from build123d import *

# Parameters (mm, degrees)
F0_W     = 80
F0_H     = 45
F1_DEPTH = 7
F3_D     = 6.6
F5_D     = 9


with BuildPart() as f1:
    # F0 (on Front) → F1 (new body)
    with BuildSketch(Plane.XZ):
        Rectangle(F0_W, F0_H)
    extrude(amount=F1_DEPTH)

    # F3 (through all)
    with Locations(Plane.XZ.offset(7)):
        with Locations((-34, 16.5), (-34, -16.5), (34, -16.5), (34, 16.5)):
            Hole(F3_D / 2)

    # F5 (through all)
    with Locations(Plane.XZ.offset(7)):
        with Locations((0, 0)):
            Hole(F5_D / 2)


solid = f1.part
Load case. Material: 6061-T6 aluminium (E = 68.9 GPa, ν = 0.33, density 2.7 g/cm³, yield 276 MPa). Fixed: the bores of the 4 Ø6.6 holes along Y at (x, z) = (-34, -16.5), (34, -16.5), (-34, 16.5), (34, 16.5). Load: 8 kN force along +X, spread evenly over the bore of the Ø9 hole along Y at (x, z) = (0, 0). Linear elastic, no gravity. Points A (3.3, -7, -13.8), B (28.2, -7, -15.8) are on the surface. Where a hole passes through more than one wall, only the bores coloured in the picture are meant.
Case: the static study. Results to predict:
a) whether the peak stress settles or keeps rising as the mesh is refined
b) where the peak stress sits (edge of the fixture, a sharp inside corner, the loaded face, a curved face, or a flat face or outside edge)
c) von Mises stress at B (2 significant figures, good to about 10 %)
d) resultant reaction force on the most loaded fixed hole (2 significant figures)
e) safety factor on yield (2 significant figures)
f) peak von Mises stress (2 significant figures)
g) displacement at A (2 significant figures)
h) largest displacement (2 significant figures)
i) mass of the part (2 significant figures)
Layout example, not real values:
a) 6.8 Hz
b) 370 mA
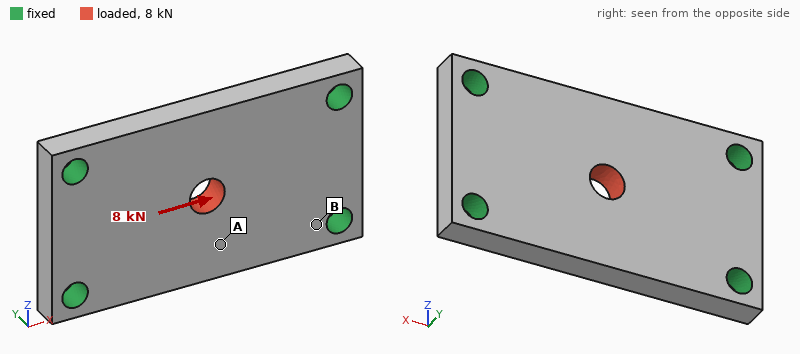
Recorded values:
a) settles
b) the loaded face
c) 23 MPa
d) 2.1 kN
e) 4.0
f) 69 MPa
g) 5.0 µm
h) 11 µm
i) 64 g
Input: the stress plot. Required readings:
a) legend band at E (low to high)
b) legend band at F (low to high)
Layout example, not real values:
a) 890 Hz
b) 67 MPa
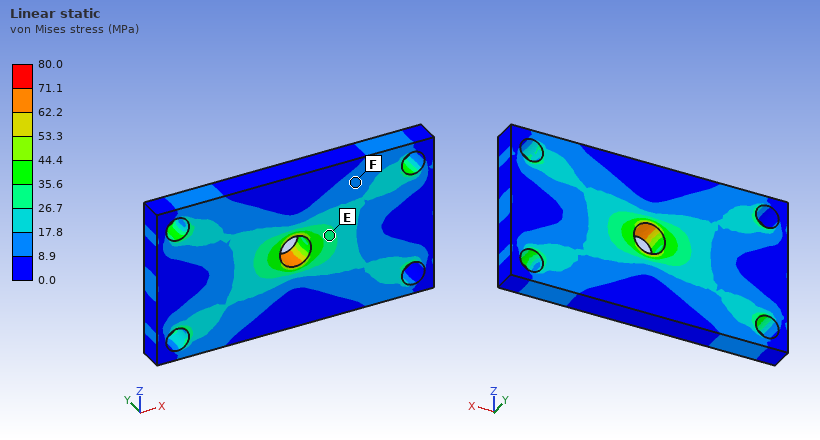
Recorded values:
a) 26.7 to 35.6 MPa
b) 8.9 to 17.8 MPa
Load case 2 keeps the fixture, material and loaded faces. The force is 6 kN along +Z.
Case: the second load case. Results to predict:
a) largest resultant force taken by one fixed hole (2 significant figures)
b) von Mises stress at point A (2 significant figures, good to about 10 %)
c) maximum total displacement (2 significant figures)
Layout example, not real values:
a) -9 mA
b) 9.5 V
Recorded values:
a) 2.1 kN
b) 14 MPa
c) 17 µm
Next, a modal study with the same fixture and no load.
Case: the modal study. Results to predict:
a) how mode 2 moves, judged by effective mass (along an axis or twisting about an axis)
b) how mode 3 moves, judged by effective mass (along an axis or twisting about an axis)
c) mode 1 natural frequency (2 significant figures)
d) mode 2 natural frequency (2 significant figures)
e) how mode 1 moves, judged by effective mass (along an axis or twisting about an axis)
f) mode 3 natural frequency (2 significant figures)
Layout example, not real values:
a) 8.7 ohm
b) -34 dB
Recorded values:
a) twisting about X
b) twisting about Z
c) 7500 Hz
d) 11 kHz
e) along Y
f) 19 kHz
